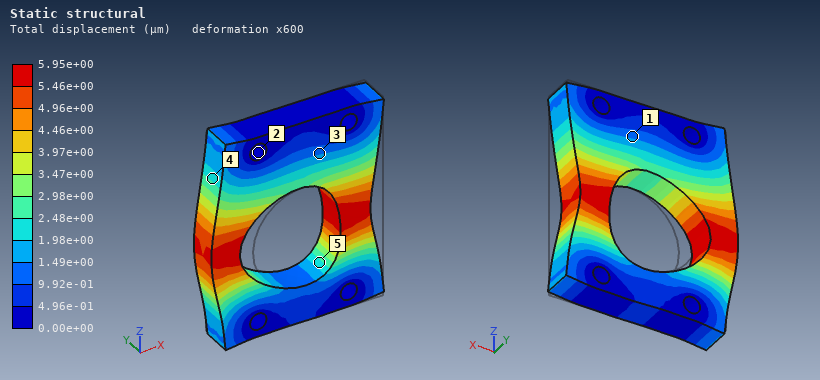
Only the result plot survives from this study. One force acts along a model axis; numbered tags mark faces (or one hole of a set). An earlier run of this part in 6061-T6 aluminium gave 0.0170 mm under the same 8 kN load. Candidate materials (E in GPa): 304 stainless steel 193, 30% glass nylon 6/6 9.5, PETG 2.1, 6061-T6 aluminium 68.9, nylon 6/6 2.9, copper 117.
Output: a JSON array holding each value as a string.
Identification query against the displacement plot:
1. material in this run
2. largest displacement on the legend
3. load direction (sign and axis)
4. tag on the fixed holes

["304 stainless steel", "5.95e+00 µm", "-X", "2"]
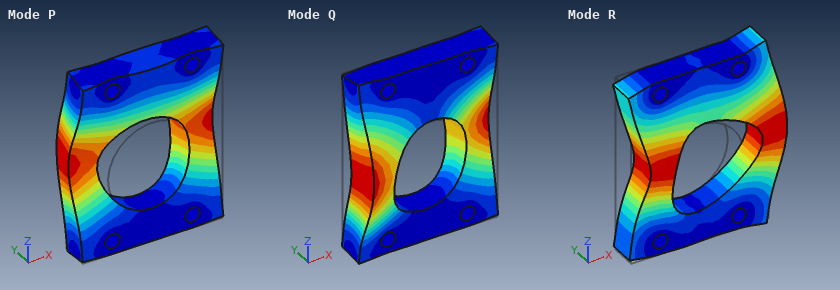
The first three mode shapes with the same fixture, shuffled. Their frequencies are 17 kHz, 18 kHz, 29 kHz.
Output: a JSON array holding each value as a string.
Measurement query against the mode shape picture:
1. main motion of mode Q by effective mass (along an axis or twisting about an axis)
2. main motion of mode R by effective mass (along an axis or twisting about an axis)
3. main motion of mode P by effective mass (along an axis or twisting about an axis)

["twisting about Z", "along X", "along Y"]
